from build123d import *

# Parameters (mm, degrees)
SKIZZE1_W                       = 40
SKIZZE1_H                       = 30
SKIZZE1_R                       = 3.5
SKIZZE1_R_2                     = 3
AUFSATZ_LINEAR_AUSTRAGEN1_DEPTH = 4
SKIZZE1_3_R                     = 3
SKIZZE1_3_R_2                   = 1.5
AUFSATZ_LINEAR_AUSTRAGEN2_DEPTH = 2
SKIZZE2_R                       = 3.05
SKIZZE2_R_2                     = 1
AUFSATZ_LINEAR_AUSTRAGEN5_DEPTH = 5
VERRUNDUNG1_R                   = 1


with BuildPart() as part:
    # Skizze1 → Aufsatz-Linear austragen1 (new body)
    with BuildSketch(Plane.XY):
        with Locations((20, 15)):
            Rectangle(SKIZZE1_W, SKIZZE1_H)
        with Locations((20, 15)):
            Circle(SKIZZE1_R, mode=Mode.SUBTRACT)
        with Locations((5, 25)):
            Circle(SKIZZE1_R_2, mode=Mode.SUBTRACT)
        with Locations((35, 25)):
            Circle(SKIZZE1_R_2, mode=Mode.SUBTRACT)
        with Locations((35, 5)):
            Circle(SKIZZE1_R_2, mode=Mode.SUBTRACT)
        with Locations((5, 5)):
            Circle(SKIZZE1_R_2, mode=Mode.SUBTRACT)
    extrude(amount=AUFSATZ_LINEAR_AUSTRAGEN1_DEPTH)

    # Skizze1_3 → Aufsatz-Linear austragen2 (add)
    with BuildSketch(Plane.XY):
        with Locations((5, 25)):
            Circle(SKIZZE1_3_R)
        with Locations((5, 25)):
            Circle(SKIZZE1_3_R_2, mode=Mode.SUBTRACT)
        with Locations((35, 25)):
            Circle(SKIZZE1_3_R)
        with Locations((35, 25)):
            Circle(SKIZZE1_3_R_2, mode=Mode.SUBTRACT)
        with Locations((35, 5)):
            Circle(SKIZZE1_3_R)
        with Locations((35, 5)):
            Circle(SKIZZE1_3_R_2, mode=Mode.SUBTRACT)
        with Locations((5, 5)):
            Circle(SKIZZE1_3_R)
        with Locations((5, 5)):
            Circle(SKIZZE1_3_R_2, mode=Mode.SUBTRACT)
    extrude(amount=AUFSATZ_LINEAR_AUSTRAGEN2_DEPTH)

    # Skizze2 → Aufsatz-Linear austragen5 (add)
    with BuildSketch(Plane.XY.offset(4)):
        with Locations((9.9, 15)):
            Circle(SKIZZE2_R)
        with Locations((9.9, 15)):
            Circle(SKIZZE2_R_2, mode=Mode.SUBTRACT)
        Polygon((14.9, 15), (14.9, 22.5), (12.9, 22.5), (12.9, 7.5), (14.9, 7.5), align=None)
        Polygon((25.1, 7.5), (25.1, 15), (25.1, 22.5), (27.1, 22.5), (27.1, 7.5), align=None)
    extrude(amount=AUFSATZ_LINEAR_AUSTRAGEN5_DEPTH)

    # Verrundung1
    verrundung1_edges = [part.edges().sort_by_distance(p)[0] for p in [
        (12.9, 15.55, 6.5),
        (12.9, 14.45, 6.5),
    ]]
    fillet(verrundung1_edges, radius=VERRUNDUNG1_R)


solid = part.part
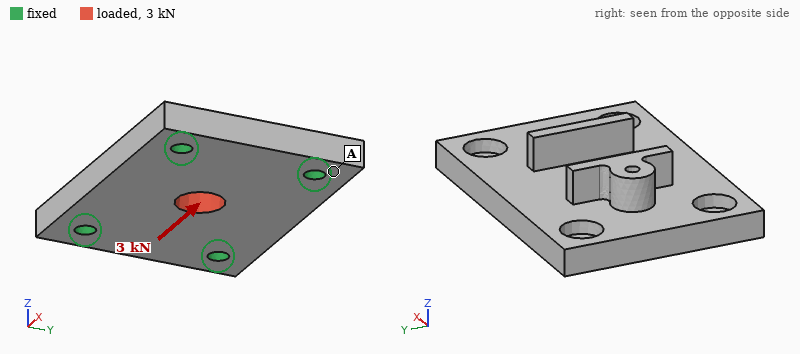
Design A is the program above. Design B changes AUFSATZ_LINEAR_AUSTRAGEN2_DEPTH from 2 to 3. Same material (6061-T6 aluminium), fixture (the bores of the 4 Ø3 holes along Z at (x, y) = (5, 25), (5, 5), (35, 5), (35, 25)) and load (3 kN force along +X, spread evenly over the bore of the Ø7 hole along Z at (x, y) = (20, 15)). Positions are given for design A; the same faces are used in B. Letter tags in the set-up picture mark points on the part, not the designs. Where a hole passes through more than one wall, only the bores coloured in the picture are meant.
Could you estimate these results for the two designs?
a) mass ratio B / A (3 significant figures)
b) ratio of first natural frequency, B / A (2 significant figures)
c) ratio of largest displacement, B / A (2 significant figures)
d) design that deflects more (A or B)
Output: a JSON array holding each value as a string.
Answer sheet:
["1.02", "1.1", "0.86", "A"]
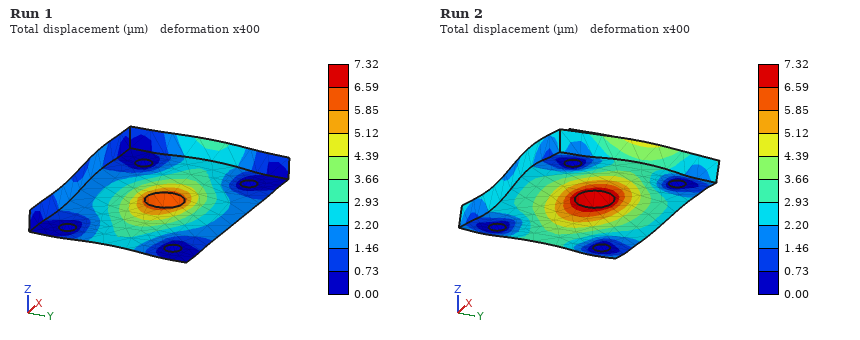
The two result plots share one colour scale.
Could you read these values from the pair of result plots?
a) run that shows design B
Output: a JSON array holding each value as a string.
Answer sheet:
["Run 1"]
